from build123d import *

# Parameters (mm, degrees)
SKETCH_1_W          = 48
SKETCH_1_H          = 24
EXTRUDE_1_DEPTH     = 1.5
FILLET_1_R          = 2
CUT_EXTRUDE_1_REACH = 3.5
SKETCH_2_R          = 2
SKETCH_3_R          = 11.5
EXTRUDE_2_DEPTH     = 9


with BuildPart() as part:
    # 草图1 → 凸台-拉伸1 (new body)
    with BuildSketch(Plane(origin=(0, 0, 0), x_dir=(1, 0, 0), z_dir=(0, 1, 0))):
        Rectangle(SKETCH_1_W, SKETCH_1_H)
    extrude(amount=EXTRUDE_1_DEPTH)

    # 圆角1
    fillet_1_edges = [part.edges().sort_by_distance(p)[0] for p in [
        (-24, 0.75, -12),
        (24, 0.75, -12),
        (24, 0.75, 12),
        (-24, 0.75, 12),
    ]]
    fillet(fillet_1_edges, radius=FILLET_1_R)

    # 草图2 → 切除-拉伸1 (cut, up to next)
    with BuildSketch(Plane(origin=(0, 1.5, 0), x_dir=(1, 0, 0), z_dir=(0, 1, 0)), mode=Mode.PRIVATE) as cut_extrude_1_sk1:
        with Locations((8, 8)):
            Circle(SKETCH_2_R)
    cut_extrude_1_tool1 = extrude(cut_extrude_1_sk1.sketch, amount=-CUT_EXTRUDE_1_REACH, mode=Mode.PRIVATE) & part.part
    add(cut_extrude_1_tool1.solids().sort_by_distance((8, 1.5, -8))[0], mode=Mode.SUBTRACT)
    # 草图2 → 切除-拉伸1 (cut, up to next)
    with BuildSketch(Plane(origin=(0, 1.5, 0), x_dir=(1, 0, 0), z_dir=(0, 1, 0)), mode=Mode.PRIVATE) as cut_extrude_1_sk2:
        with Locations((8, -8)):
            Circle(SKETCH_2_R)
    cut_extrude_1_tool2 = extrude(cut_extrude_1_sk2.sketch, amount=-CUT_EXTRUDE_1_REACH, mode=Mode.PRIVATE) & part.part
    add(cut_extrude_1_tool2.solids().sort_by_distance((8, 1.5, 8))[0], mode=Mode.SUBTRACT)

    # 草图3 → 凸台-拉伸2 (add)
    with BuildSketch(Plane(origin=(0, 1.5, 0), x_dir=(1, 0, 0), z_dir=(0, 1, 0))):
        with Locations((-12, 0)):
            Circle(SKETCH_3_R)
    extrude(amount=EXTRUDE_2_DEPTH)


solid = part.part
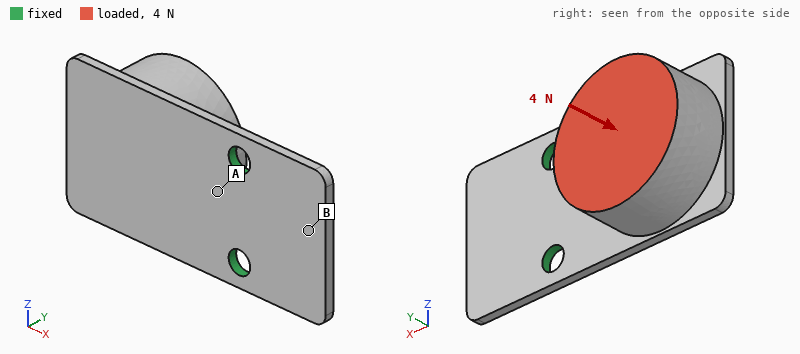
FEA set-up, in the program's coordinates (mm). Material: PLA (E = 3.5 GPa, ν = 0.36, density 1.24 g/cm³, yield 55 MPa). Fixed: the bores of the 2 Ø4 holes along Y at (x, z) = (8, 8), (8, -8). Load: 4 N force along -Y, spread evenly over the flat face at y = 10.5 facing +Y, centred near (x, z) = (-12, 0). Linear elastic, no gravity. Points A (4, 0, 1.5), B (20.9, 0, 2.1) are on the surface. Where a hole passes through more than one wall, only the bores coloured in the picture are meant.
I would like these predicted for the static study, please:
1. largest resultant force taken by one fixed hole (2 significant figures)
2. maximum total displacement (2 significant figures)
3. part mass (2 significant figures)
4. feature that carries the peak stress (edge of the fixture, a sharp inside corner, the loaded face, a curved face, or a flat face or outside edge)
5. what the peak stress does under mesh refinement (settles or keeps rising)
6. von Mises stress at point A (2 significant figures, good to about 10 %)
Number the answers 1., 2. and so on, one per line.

1. 2.1 N
2. 0.55 mm
3. 6.7 g
4. edge of the fixture
5. keeps rising
6. 4.9 MPa
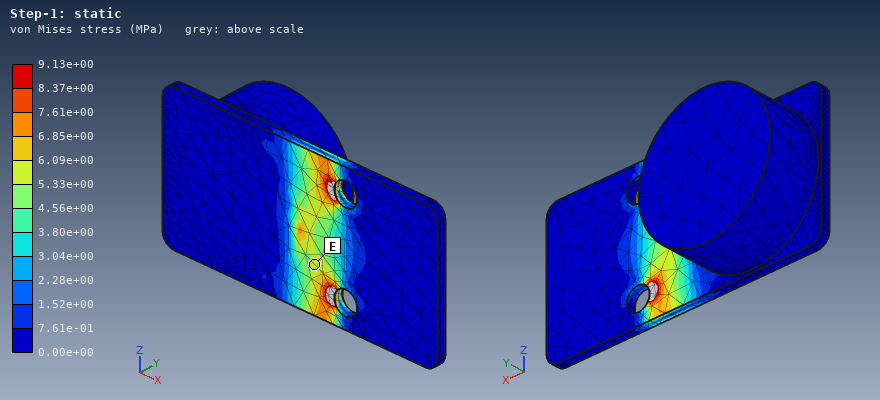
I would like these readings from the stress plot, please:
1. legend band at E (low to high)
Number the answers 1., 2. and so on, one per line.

1. 5.33e+00 to 6.09e+00 MPa
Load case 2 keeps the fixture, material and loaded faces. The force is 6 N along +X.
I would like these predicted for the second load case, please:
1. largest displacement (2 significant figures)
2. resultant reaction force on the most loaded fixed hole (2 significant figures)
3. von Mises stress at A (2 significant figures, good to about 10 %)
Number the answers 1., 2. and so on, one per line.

1. 0.55 mm
2. 3.2 N
3. 4.7 MPa
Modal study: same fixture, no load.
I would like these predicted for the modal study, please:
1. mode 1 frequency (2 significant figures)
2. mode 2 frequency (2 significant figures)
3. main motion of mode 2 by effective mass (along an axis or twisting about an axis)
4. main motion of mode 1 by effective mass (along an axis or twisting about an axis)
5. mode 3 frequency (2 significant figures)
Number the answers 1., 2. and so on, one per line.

1. 220 Hz
2. 1000 Hz
3. along Z
4. along Y
5. 1900 Hz
